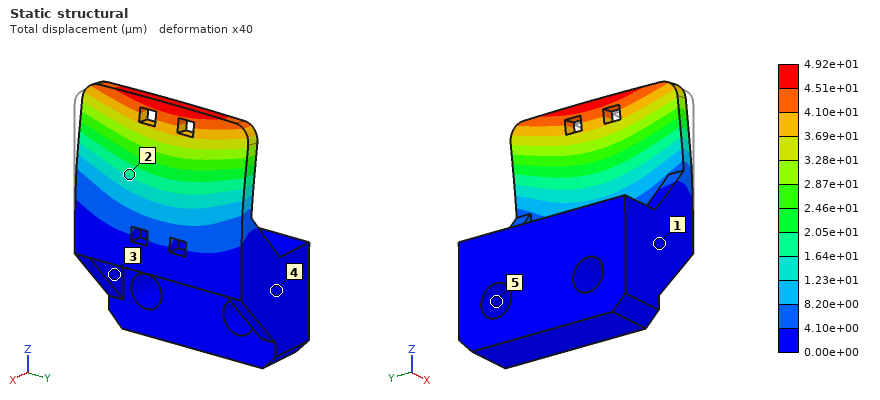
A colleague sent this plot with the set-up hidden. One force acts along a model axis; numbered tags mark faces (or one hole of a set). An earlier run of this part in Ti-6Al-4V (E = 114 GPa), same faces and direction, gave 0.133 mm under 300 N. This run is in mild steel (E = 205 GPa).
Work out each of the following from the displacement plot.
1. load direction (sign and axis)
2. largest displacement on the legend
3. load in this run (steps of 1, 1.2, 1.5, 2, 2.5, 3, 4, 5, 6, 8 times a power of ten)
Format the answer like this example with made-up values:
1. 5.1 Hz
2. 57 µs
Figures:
1. -X
2. 4.92e+01 µm
3. 200 N
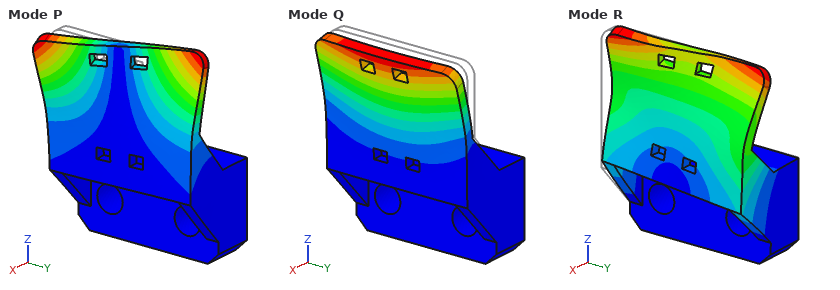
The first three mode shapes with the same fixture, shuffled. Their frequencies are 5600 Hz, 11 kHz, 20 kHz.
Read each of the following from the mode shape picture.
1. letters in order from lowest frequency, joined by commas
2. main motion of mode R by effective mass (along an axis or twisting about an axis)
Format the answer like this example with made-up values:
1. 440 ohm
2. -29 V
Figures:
1. Q, P, R
2. along Y
